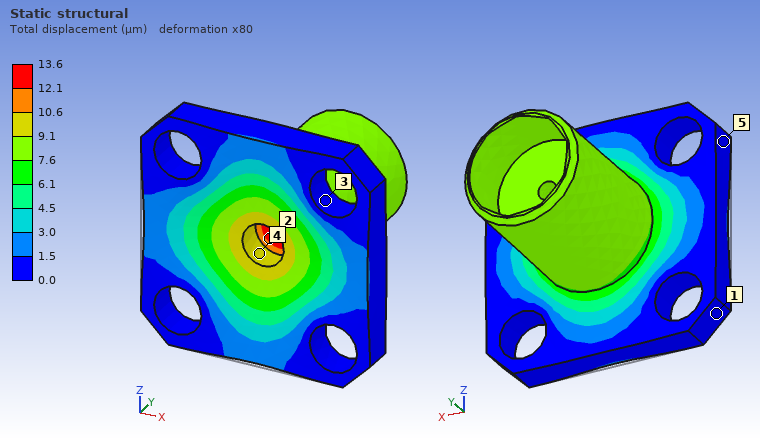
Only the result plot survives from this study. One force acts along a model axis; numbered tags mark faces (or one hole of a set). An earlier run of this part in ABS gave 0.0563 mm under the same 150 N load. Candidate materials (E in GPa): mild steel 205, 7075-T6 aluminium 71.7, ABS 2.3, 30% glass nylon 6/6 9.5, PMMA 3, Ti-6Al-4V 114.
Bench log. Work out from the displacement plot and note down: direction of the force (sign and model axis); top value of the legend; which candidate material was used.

+Y
13.6 µm
30% glass nylon 6/6
